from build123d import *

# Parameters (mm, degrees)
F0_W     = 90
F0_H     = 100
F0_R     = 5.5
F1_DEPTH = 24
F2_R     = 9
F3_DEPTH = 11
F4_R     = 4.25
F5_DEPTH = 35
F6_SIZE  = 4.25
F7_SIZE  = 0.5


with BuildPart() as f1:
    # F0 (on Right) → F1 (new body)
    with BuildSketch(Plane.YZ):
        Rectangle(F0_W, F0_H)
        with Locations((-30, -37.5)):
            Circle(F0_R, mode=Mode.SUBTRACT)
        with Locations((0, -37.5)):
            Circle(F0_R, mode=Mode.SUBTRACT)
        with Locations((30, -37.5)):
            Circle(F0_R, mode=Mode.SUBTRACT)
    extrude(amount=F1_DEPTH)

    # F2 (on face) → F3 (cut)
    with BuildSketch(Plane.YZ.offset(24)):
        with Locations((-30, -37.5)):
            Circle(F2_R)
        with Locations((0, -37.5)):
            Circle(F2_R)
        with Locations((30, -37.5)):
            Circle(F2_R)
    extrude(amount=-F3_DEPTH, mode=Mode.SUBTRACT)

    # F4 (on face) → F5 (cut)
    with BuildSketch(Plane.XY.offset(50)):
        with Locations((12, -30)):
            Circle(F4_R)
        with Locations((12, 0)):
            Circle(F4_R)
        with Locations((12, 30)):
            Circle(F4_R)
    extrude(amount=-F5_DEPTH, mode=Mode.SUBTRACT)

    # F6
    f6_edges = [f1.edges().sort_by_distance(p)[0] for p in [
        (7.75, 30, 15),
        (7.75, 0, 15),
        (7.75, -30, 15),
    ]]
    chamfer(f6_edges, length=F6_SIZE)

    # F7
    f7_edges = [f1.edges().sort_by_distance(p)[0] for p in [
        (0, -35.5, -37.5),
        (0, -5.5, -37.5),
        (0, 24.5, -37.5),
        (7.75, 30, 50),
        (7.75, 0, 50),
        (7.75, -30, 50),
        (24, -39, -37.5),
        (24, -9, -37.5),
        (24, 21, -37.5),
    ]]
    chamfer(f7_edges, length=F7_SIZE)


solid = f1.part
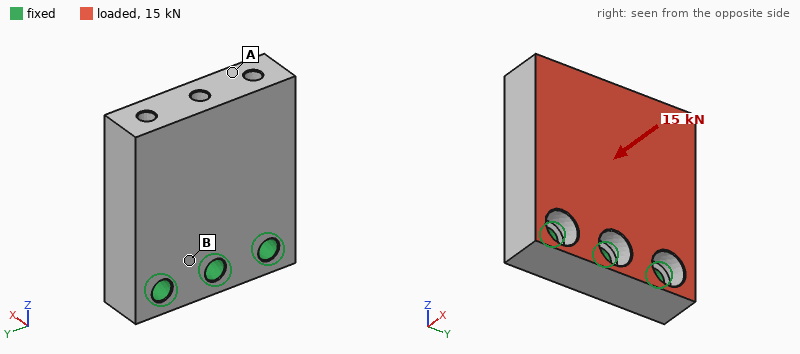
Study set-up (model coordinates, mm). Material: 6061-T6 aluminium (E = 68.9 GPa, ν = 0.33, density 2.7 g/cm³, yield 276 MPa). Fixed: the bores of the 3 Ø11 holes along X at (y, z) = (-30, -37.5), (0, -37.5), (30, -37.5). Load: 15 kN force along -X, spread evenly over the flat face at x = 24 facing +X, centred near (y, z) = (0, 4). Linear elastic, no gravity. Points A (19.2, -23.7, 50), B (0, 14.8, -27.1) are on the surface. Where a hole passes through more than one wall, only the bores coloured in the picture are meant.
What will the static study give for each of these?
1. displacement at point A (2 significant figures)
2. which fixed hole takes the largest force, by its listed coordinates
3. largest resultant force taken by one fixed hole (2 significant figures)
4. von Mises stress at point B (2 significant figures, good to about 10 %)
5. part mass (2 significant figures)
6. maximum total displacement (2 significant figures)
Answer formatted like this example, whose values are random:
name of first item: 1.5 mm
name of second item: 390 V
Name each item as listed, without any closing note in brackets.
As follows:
displacement at point A: 0.34 mm
which fixed hole takes the largest force, by its listed coordinates: (0, -37.5)
largest resultant force taken by one fixed hole: 6.0 kN
von Mises stress at point B: 60 MPa
part mass: 540 g
maximum total displacement: 0.34 mm
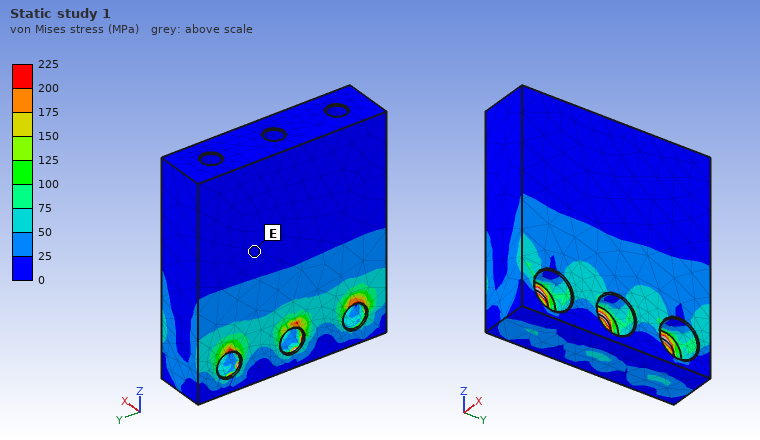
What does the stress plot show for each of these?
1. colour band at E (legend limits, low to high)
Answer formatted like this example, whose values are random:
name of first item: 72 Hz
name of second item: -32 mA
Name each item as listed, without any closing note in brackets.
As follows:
colour band at E: 0 to 25 MPa
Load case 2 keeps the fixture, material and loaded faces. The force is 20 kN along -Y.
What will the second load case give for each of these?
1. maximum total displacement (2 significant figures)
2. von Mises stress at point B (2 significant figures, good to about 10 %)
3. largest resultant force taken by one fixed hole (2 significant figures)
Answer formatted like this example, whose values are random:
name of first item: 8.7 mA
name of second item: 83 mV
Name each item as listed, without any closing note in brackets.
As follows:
maximum total displacement: 68 µm
von Mises stress at point B: 17 MPa
largest resultant force taken by one fixed hole: 15 kN
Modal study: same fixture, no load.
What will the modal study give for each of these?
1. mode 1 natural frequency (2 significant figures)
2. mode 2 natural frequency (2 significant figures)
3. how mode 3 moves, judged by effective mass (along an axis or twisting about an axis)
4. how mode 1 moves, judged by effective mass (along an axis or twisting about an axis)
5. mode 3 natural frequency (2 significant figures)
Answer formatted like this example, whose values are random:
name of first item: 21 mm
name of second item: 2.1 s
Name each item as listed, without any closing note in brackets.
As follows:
mode 1 natural frequency: 1800 Hz
mode 2 natural frequency: 4500 Hz
how mode 3 moves, judged by effective mass: along Y
how mode 1 moves, judged by effective mass: along X
mode 3 natural frequency: 5500 Hz
